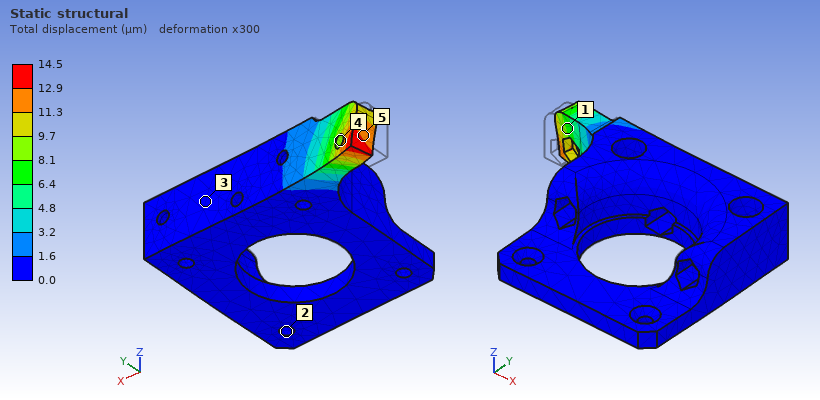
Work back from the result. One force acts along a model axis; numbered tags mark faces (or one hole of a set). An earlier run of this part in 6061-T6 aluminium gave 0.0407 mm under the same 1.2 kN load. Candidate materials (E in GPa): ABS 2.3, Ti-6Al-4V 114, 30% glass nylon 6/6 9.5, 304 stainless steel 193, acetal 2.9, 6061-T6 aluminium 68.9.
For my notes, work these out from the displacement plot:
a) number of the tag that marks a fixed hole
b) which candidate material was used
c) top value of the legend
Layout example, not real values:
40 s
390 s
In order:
2
304 stainless steel
14.5 µm
